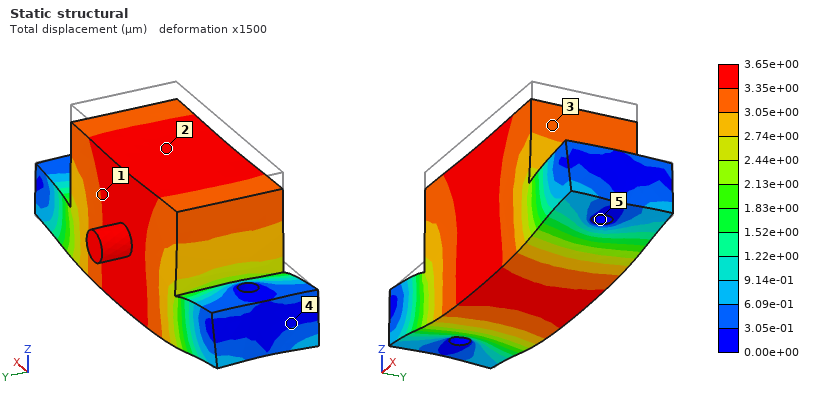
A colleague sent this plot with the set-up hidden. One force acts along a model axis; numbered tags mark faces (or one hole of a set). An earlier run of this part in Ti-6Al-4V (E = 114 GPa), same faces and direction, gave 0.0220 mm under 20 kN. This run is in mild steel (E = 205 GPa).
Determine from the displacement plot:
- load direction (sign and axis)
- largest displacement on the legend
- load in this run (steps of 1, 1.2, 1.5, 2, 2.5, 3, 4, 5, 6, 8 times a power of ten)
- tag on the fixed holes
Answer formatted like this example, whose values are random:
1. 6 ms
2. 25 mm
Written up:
1. -Z
2. 3.65e+00 µm
3. 6 kN
4. 5
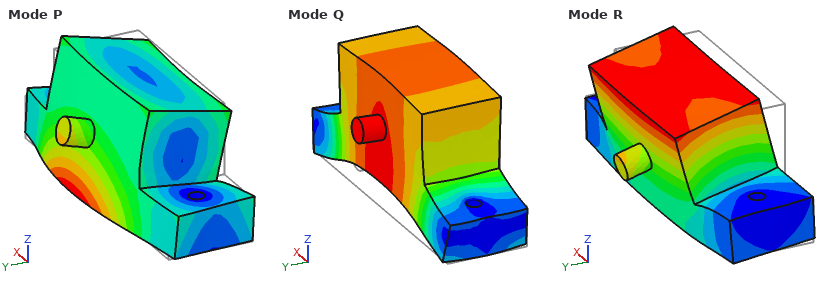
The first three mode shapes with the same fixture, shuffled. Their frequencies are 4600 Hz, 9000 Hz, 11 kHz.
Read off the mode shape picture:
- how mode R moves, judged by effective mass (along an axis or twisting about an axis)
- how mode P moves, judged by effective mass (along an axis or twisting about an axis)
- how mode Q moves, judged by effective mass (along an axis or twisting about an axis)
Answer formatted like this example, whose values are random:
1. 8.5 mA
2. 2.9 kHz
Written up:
1. along Y
2. along Y
3. along Z
